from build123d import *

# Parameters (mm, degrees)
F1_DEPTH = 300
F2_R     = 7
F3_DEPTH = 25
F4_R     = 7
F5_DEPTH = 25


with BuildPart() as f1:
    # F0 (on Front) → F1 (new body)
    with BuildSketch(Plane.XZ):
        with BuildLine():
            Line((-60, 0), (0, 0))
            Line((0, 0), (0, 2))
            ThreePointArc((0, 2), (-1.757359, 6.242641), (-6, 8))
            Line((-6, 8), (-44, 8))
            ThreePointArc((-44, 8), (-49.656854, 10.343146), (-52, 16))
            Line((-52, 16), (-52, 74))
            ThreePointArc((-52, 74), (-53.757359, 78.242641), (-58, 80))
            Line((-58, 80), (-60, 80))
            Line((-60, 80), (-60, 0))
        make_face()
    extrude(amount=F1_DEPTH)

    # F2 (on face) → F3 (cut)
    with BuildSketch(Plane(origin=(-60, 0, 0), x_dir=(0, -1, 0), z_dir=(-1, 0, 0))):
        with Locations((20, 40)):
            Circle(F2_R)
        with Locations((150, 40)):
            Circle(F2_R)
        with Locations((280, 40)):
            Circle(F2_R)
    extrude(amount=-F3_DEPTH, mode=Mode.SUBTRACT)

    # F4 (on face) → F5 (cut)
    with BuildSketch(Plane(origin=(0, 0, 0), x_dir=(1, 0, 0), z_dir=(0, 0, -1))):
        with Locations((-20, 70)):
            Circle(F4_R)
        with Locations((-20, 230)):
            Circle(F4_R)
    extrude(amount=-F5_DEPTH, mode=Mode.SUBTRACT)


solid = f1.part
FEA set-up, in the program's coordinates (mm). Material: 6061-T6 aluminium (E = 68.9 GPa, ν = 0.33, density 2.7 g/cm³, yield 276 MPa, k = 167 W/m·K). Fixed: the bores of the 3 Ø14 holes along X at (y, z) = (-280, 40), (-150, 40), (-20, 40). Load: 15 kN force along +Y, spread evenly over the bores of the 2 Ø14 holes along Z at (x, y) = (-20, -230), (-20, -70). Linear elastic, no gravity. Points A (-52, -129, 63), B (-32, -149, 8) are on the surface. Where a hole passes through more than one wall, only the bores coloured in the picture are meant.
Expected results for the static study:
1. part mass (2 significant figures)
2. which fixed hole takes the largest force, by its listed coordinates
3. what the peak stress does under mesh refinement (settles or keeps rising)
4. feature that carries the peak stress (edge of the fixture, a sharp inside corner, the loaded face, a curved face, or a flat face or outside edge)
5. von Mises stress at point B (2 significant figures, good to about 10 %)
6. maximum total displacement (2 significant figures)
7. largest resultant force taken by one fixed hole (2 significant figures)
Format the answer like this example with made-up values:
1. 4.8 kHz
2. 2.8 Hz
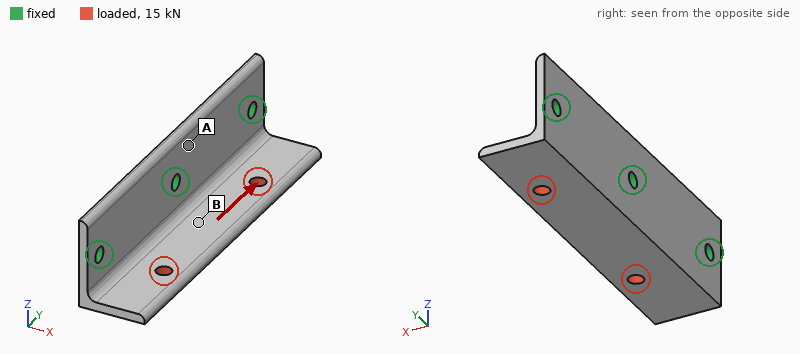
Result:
1. 840 g
2. (-150, 40)
3. keeps rising
4. edge of the fixture
5. 19 MPa
6. 0.27 mm
7. 6.7 kN
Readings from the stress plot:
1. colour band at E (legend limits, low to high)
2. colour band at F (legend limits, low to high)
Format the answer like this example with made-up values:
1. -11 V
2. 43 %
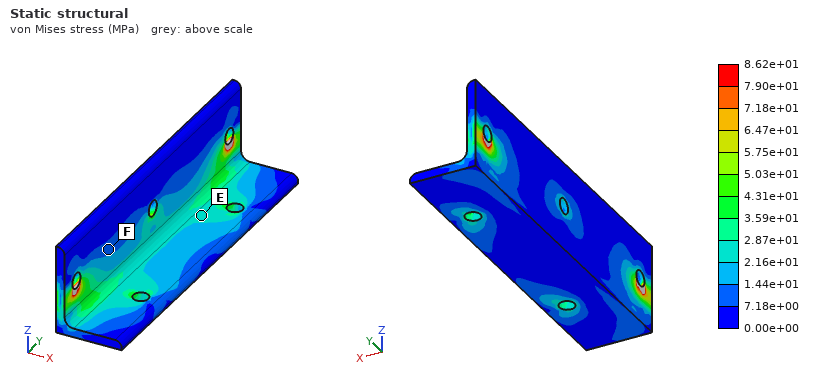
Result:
1. 2.16e+01 to 2.87e+01 MPa
2. 7.18e+00 to 1.44e+01 MPa
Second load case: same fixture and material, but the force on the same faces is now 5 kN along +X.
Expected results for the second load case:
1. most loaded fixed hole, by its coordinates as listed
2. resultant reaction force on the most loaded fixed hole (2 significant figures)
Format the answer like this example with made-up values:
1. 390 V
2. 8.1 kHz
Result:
1. (-150, 40)
2. 2.1 kN
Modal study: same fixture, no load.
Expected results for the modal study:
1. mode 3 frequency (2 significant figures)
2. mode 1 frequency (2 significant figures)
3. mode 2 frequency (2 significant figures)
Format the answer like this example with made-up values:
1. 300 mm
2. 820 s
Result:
1. 2400 Hz
2. 1000 Hz
3. 1300 Hz
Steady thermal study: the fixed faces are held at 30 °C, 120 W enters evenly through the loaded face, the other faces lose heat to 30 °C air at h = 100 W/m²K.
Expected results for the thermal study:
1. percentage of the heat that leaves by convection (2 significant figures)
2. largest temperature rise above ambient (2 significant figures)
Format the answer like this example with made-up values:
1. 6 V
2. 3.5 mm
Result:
1. 52 %
2. 28 K
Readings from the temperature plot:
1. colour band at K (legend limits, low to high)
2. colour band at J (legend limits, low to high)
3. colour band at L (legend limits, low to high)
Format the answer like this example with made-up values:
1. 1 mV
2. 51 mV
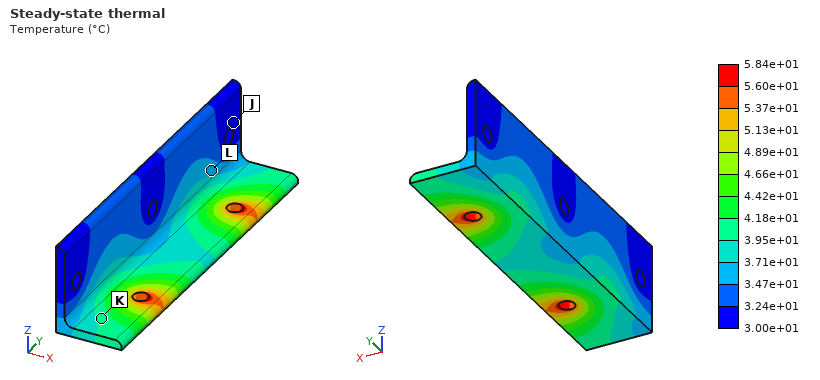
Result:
1. 3.95e+01 to 4.18e+01 °C
2. 3.00e+01 to 3.24e+01 °C
3. 3.47e+01 to 3.71e+01 °C
